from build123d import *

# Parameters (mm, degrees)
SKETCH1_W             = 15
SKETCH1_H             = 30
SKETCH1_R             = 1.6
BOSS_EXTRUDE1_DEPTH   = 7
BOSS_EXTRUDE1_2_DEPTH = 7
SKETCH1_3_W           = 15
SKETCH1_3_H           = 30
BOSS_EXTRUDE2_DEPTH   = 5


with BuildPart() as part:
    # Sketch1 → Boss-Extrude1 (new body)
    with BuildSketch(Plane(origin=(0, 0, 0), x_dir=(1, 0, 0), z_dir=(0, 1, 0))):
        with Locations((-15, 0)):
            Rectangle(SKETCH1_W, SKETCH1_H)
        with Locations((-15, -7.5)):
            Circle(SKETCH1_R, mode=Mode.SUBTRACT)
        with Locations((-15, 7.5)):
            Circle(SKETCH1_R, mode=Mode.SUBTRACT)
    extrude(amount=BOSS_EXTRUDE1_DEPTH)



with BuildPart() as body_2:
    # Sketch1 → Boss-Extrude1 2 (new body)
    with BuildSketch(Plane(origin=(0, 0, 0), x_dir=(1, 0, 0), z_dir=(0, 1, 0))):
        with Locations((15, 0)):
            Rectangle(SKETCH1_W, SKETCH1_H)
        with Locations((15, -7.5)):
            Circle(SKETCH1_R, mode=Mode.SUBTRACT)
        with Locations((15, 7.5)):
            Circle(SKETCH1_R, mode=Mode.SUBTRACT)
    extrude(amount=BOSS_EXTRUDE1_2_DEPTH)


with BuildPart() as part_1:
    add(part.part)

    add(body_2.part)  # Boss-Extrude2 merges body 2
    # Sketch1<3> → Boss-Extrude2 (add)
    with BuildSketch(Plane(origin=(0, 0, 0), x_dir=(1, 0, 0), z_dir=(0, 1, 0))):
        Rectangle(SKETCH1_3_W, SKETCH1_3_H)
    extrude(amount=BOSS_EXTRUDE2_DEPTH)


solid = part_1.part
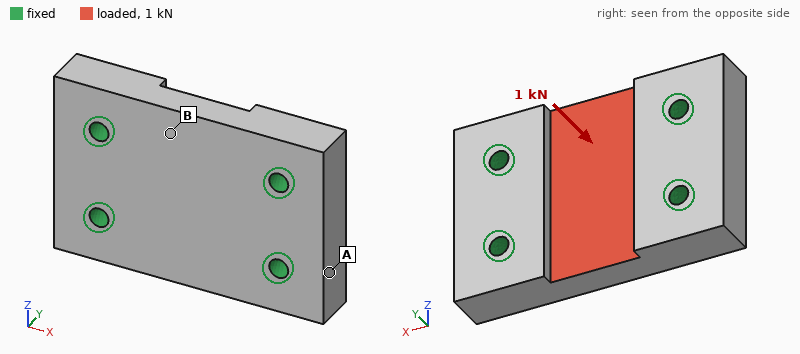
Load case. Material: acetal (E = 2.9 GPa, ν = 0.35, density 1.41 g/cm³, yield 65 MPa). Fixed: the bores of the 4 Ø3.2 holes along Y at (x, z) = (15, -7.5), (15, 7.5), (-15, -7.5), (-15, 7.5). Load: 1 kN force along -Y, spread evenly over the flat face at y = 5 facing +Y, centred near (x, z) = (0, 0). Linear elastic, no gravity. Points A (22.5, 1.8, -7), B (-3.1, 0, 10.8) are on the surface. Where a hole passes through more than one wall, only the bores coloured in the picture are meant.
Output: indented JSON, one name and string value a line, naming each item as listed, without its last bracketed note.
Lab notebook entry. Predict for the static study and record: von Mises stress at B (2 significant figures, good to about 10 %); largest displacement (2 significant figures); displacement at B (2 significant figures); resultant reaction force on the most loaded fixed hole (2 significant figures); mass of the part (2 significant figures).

{
  "von Mises stress at B": "11 MPa",
  "largest displacement": "0.12 mm",
  "displacement at B": "0.098 mm",
  "resultant reaction force on the most loaded fixed hole": "260 N",
  "mass of the part": "12 g"
}
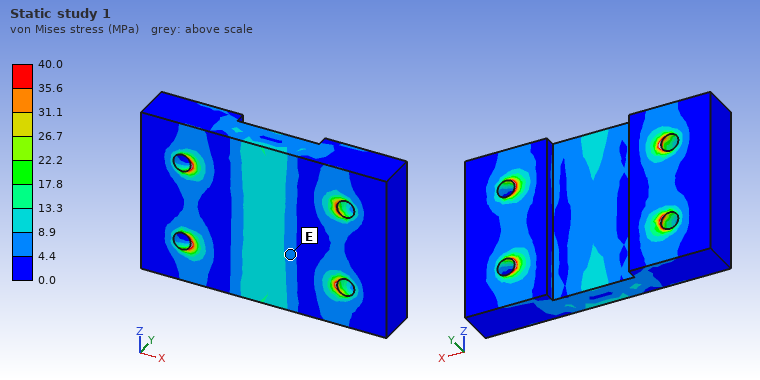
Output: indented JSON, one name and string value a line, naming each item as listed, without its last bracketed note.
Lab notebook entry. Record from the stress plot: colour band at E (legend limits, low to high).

{
  "colour band at E": "4.4 to 8.9 MPa"
}
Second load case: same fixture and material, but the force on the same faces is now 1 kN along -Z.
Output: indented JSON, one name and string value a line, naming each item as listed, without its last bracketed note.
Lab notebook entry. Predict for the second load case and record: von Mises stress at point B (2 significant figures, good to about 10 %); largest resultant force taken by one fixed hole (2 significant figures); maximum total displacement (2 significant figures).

{
  "von Mises stress at point B": "4.1 MPa",
  "largest resultant force taken by one fixed hole": "280 N",
  "maximum total displacement": "68 µm"
}
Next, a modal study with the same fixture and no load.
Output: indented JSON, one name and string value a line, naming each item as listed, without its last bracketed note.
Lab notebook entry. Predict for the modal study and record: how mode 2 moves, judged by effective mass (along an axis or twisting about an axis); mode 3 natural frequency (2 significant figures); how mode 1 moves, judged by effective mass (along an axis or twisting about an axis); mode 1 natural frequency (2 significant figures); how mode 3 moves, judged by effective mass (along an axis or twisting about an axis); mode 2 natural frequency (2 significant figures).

{
  "how mode 2 moves, judged by effective mass": "twisting about X",
  "mode 3 natural frequency": "13 kHz",
  "how mode 1 moves, judged by effective mass": "along Y",
  "mode 1 natural frequency": "8400 Hz",
  "how mode 3 moves, judged by effective mass": "along Z",
  "mode 2 natural frequency": "9400 Hz"
}
